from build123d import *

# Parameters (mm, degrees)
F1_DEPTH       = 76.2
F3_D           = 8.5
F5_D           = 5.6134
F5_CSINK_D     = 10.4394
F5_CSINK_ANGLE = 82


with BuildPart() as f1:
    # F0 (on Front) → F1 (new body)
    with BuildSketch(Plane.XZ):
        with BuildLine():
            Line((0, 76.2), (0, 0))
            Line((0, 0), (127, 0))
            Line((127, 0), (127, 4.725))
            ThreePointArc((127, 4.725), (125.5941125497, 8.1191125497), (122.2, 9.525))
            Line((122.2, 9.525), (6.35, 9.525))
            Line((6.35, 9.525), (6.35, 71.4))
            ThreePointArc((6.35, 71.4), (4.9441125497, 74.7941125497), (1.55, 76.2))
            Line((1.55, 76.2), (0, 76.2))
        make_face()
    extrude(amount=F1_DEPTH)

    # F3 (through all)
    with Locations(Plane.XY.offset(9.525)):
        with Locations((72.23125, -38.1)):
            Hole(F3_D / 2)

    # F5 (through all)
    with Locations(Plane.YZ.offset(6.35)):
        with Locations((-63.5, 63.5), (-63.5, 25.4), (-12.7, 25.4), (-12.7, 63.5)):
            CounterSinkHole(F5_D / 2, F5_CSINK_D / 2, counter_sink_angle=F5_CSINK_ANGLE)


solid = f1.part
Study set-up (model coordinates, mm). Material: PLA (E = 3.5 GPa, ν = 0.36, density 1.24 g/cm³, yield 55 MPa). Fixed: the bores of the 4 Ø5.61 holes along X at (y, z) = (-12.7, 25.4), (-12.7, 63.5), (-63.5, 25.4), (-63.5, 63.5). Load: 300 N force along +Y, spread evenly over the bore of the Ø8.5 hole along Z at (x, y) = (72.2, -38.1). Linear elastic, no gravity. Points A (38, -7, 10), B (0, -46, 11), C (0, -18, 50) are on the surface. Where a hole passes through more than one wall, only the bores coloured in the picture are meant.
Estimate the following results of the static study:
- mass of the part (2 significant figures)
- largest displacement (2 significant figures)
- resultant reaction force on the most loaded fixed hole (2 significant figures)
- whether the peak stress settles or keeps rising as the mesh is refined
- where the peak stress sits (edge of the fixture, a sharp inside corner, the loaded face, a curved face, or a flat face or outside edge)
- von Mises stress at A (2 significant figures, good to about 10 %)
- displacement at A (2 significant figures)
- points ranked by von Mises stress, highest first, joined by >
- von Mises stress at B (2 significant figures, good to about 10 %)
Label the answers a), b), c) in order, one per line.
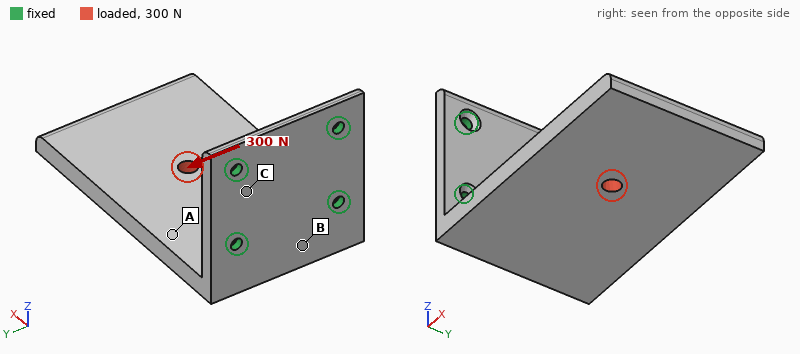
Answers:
a) 150 g
b) 1.4 mm
c) 480 N
d) keeps rising
e) edge of the fixture
f) 2.8 MPa
g) 0.53 mm
h) B > A > C
i) 6.1 MPa
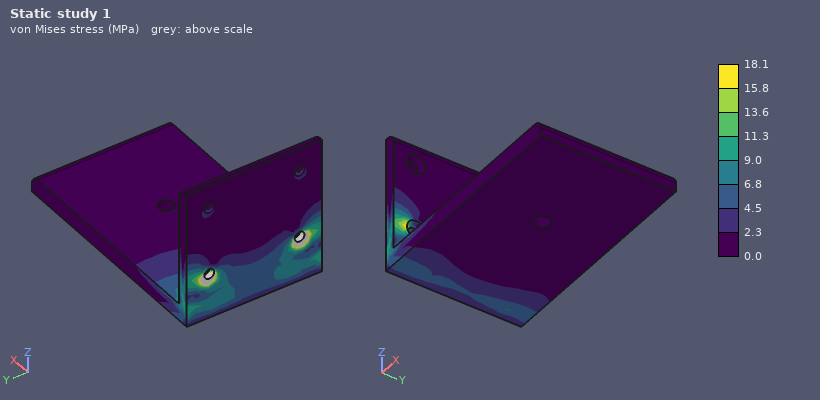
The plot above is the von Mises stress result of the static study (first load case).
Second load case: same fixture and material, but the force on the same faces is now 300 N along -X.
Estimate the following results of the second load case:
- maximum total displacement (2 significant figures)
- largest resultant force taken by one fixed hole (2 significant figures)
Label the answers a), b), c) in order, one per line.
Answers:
a) 1.9 mm
b) 210 N
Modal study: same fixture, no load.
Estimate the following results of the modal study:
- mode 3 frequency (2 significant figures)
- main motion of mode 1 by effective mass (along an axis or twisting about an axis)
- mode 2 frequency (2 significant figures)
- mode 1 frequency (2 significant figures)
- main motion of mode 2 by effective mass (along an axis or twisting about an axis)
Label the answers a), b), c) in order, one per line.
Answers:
a) 550 Hz
b) along Z
c) 280 Hz
d) 93 Hz
e) along Y
